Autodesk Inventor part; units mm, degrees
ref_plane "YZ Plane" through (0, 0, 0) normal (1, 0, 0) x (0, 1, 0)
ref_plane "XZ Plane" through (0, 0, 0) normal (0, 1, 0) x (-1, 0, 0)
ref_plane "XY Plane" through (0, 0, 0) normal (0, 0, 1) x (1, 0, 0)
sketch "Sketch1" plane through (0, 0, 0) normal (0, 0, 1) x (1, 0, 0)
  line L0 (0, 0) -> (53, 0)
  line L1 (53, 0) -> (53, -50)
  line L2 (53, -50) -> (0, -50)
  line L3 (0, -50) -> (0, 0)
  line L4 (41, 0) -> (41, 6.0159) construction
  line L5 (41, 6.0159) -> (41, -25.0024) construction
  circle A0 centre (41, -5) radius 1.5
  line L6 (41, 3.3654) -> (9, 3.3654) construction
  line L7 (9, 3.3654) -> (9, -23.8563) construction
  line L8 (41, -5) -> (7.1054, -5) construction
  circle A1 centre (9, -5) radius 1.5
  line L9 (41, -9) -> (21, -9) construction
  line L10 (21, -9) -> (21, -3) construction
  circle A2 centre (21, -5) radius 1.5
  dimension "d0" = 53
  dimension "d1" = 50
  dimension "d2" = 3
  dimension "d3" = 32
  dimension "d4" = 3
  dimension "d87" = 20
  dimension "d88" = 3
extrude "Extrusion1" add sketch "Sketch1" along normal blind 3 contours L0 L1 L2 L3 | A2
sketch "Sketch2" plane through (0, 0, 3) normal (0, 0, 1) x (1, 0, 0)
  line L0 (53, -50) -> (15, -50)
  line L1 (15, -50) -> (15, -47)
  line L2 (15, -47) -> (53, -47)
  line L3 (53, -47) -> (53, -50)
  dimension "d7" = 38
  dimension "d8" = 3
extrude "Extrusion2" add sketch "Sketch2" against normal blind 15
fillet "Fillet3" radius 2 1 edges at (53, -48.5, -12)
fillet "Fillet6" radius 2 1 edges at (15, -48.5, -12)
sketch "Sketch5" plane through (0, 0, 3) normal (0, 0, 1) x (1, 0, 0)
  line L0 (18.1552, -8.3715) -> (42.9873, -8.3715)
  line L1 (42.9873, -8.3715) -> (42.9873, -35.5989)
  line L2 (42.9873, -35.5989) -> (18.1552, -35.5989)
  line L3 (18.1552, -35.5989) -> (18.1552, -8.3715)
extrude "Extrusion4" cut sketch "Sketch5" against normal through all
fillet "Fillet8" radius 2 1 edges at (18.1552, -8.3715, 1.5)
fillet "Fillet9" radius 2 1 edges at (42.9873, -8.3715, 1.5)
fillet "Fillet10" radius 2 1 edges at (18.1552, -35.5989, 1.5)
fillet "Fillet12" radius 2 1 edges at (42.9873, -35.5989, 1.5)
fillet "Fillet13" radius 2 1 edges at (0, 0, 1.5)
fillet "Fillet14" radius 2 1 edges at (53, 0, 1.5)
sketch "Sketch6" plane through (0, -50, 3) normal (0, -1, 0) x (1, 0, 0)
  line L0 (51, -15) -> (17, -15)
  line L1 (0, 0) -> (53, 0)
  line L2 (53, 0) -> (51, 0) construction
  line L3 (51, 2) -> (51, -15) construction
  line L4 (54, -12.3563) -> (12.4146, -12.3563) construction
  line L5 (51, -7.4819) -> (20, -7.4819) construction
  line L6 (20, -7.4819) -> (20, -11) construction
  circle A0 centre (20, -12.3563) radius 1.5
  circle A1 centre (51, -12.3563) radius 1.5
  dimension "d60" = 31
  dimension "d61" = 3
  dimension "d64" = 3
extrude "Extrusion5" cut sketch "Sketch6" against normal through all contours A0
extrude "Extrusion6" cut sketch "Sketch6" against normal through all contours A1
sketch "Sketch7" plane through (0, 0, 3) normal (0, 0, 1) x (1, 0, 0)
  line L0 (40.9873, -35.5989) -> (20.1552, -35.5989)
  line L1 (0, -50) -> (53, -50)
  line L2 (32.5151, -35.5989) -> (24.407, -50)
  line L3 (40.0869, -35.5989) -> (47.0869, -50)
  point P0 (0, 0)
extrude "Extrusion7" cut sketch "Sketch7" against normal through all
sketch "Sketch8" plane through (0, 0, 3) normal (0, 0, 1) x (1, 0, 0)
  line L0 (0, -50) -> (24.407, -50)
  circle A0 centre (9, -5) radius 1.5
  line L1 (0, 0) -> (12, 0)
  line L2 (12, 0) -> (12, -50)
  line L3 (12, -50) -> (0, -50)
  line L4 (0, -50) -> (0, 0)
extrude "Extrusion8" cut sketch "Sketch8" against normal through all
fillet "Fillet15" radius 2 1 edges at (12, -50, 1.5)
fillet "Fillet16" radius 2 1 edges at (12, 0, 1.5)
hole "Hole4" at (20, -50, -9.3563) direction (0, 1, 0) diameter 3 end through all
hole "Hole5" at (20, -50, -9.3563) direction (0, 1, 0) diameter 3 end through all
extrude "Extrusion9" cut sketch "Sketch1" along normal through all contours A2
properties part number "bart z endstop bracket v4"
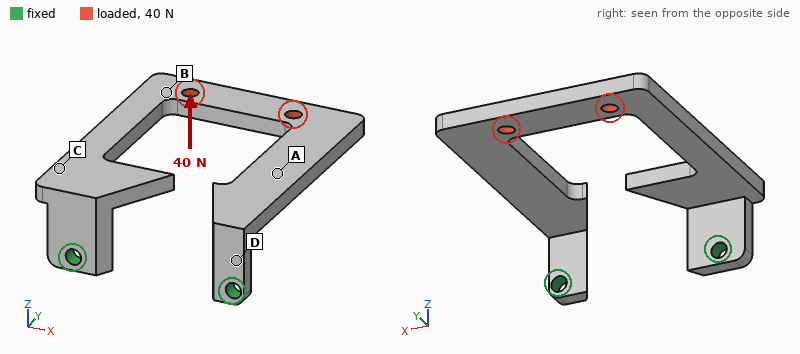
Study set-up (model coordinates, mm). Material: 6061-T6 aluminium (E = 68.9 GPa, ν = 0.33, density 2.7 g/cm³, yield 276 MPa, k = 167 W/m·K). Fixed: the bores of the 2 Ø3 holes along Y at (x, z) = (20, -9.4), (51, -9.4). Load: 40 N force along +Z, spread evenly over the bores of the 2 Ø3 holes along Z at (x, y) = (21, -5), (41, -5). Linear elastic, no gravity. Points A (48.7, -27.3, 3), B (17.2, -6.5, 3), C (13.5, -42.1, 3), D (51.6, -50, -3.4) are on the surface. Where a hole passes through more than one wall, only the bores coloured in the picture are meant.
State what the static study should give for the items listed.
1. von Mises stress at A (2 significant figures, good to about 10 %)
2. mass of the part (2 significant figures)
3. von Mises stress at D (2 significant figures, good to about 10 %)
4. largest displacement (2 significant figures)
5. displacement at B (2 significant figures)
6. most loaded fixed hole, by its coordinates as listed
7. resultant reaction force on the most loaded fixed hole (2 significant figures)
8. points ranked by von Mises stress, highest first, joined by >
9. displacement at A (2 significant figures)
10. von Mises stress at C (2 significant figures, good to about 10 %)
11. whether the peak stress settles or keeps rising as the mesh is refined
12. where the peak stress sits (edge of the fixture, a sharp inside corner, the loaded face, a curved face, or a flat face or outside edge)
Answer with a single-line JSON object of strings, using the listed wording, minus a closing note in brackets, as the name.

{"von Mises stress at A": "29 MPa", "mass of the part": "11 g", "von Mises stress at D": "81 MPa", "largest displacement": "0.79 mm", "displacement at B": "0.63 mm", "most loaded fixed hole, by its coordinates as listed": "(20, -9.4)", "resultant reaction force on the most loaded fixed hole": "23 N", "points ranked by von Mises stress, highest first, joined by >": "D > C > A > B", "displacement at A": "0.27 mm", "von Mises stress at C": "42 MPa", "whether the peak stress settles or keeps rising as the mesh is refined": "keeps rising", "where the peak stress sits": "edge of the fixture"}
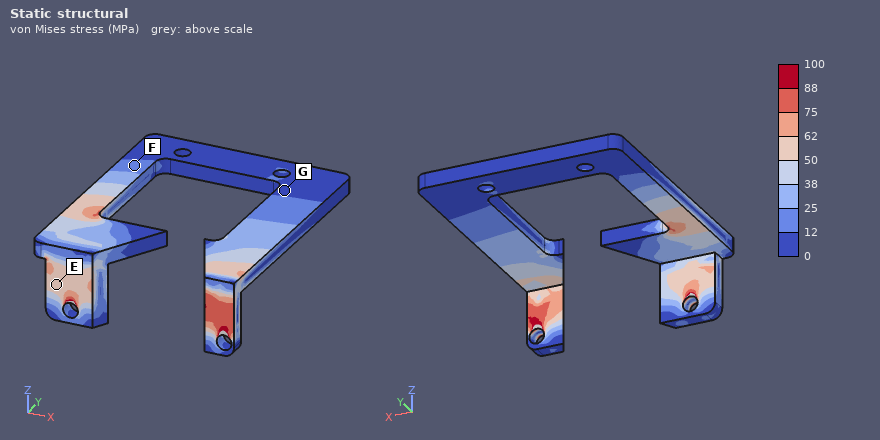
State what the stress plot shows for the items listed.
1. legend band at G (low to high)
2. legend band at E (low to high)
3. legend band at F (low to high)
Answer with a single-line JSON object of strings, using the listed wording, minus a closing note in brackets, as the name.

{"legend band at G": "0 to 12 MPa", "legend band at E": "50 to 62 MPa", "legend band at F": "12 to 25 MPa"}
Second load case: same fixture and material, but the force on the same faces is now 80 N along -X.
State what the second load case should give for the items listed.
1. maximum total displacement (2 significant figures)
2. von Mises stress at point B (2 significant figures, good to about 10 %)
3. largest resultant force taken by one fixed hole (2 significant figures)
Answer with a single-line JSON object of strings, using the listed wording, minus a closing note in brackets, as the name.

{"maximum total displacement": "0.17 mm", "von Mises stress at point B": "15 MPa", "largest resultant force taken by one fixed hole": "87 N"}
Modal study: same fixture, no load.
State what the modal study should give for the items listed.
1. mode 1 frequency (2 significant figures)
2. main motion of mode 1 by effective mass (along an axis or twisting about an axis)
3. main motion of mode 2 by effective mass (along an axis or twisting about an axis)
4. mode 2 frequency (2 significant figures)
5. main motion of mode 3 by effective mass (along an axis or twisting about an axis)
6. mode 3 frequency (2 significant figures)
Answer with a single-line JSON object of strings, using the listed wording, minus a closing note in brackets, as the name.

{"mode 1 frequency": "610 Hz", "main motion of mode 1 by effective mass": "along Z", "main motion of mode 2 by effective mass": "along X", "mode 2 frequency": "1600 Hz", "main motion of mode 3 by effective mass": "along X", "mode 3 frequency": "1900 Hz"}
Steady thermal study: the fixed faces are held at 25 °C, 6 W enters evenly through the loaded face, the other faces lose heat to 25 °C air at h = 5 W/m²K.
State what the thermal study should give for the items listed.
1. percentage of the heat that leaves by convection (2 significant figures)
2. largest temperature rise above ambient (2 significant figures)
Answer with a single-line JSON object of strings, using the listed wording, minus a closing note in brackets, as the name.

{"percentage of the heat that leaves by convection": "6.1 %", "largest temperature rise above ambient": "40 K"}
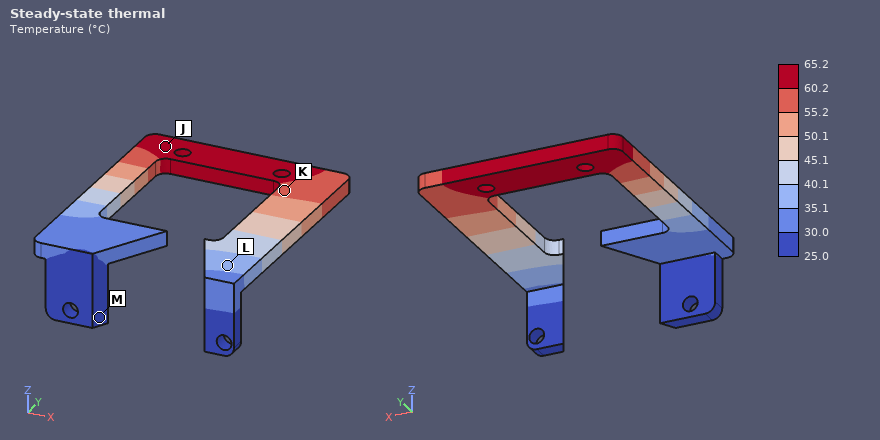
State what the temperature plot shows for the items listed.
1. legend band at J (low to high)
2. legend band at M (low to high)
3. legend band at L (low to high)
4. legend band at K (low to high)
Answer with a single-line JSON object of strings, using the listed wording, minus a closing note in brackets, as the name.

{"legend band at J": "60.2 to 65.2 °C", "legend band at M": "25.0 to 30.0 °C", "legend band at L": "35.1 to 40.1 °C", "legend band at K": "55.2 to 60.2 °C"}
